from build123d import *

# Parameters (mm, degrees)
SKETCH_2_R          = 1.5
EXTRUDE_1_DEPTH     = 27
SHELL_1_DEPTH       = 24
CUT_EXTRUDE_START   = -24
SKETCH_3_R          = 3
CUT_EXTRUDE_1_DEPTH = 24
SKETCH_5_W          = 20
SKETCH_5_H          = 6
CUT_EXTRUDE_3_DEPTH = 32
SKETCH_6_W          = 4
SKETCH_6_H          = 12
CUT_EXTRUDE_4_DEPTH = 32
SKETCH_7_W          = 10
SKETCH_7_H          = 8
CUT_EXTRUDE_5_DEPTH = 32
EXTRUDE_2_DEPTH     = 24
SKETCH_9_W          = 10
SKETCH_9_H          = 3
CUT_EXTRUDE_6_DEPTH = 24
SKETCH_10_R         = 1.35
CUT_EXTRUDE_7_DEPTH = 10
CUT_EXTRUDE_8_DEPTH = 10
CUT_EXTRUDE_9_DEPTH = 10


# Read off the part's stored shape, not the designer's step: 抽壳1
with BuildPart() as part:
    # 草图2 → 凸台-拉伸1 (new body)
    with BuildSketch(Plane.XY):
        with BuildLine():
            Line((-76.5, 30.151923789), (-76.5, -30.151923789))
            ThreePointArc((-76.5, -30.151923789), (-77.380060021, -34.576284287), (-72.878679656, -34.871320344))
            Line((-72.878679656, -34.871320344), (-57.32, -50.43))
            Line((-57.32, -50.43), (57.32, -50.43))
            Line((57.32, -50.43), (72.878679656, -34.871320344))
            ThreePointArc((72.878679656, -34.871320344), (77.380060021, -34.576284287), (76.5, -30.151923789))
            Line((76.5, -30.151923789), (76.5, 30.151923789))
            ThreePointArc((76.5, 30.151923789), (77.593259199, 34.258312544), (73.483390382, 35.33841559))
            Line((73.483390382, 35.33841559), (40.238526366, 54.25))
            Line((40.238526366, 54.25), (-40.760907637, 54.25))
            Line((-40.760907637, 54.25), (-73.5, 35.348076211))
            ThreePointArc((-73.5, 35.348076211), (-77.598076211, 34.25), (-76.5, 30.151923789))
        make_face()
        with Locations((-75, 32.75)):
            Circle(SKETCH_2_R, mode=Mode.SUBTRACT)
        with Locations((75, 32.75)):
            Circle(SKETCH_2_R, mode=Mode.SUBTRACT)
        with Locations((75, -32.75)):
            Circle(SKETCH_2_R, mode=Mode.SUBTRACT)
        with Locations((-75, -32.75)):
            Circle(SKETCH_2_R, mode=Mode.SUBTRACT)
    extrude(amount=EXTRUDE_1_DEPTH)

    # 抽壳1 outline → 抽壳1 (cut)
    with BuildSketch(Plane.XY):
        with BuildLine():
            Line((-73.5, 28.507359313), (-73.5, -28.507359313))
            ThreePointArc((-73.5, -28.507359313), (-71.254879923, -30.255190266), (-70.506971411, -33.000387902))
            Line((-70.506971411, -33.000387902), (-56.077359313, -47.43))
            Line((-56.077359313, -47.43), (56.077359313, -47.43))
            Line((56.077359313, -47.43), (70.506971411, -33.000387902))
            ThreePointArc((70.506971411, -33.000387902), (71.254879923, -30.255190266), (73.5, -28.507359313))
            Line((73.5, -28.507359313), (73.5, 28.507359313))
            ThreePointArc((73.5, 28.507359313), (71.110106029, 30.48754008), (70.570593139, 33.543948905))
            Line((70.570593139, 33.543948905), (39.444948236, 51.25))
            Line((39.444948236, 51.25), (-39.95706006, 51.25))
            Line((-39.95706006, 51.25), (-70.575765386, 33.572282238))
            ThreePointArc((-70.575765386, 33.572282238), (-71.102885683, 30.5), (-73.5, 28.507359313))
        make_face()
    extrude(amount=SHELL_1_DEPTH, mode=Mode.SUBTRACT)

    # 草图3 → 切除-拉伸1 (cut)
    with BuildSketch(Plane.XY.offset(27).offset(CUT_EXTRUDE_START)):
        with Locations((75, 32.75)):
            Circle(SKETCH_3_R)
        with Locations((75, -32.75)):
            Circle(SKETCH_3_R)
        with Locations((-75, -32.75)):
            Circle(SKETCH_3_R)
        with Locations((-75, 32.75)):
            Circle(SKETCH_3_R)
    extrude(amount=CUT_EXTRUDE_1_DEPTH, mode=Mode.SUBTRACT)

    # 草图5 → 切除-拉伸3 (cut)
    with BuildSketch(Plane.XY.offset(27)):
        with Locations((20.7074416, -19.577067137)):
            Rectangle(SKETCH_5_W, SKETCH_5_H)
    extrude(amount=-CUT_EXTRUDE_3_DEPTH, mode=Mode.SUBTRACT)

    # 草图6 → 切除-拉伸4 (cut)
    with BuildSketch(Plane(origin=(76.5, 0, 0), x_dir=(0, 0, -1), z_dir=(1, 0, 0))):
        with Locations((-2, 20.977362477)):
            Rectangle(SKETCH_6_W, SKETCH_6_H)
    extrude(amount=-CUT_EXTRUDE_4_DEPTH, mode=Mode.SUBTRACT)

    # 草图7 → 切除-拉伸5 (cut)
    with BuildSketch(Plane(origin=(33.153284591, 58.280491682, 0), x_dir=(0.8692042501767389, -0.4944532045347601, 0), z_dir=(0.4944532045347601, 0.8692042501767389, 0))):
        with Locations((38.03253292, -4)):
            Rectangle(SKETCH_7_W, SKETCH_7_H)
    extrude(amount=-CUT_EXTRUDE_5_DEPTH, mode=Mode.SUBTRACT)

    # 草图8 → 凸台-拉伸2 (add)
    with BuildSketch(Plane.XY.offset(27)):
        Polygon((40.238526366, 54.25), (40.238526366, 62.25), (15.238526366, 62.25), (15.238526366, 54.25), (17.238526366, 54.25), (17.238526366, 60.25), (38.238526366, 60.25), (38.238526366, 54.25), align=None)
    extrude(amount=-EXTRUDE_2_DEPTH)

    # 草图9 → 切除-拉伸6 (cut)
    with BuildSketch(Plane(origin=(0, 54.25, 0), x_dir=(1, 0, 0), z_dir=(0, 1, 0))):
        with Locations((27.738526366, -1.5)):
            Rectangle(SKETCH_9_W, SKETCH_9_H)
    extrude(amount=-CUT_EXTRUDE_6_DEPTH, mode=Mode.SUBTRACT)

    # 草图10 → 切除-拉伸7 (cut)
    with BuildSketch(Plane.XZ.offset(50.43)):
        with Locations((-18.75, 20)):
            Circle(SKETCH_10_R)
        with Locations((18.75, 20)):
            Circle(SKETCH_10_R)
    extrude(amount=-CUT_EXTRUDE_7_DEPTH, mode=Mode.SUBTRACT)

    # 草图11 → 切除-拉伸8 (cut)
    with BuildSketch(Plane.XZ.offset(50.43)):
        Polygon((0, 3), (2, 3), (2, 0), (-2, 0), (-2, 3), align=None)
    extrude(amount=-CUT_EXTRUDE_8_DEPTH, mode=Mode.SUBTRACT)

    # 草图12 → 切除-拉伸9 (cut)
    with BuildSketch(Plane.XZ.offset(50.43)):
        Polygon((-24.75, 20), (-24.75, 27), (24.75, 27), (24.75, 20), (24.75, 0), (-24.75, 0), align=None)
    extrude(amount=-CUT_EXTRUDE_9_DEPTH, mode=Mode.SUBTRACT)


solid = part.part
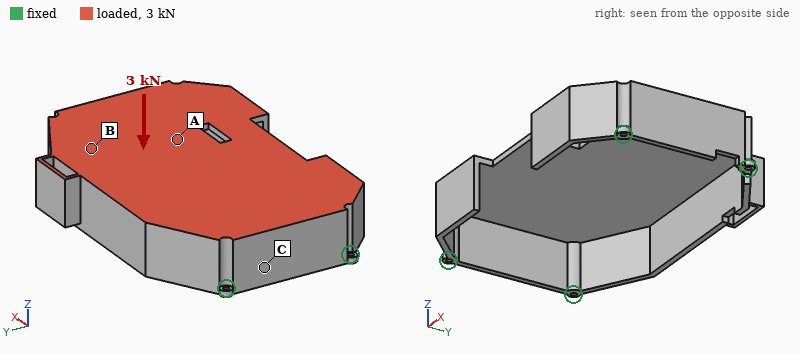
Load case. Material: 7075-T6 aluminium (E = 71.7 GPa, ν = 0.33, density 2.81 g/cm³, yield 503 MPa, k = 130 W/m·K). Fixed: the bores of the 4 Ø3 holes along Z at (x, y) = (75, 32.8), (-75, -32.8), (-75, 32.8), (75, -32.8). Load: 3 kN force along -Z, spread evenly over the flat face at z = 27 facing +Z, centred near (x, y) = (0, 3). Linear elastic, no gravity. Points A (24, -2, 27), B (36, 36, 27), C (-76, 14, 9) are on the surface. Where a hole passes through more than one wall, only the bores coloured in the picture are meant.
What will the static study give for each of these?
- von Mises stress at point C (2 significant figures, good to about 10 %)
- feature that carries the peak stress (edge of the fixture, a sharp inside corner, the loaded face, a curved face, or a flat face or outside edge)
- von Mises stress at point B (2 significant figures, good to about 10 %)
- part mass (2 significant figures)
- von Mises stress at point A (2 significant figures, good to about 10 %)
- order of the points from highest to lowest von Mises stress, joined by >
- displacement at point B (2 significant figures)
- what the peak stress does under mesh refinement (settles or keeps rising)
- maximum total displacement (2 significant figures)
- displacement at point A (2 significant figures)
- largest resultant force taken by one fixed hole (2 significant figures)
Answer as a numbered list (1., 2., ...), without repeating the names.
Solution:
1. 16 MPa
2. edge of the fixture
3. 36 MPa
4. 200 g
5. 56 MPa
6. A > B > C
7. 0.17 mm
8. keeps rising
9. 0.71 mm
10. 0.58 mm
11. 1.1 kN
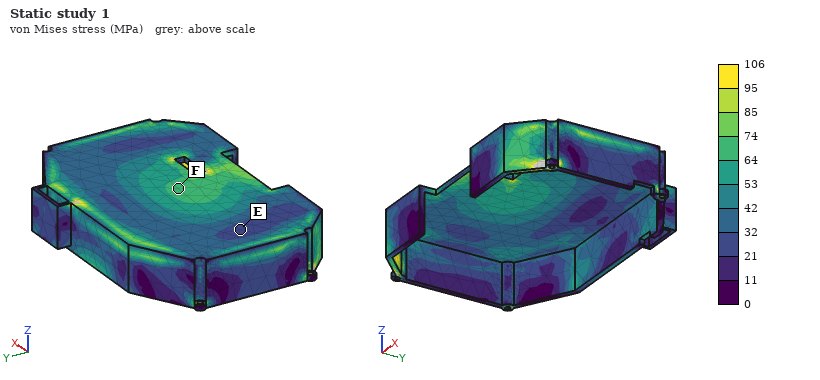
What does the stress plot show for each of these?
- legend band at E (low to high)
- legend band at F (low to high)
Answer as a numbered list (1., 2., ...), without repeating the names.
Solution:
1. 21 to 32 MPa
2. 64 to 74 MPa
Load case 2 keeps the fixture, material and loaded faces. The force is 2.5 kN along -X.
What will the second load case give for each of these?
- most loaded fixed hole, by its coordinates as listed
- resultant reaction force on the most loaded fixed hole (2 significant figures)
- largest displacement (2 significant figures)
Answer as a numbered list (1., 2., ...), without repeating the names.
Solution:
1. (-75, 32.8)
2. 1.2 kN
3. 0.30 mm
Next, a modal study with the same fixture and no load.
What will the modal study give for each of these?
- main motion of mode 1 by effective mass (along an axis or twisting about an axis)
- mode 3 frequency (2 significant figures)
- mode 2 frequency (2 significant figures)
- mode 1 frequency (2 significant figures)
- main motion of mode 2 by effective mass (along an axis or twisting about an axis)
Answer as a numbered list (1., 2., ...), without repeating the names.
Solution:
1. along Z
2. 2200 Hz
3. 1400 Hz
4. 1100 Hz
5. along X
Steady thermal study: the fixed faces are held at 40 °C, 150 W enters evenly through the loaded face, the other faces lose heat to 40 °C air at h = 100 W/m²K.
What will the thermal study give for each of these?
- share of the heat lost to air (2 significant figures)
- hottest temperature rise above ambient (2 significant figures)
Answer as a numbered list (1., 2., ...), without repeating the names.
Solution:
1. 77 %
2. 51 K
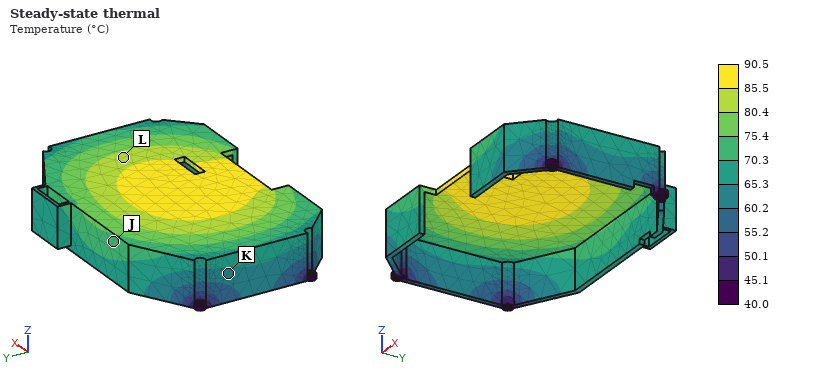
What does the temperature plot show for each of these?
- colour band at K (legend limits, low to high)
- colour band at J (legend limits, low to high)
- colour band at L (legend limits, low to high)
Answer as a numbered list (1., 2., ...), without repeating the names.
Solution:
1. 60.2 to 65.3 °C
2. 70.3 to 75.4 °C
3. 80.4 to 85.5 °C
